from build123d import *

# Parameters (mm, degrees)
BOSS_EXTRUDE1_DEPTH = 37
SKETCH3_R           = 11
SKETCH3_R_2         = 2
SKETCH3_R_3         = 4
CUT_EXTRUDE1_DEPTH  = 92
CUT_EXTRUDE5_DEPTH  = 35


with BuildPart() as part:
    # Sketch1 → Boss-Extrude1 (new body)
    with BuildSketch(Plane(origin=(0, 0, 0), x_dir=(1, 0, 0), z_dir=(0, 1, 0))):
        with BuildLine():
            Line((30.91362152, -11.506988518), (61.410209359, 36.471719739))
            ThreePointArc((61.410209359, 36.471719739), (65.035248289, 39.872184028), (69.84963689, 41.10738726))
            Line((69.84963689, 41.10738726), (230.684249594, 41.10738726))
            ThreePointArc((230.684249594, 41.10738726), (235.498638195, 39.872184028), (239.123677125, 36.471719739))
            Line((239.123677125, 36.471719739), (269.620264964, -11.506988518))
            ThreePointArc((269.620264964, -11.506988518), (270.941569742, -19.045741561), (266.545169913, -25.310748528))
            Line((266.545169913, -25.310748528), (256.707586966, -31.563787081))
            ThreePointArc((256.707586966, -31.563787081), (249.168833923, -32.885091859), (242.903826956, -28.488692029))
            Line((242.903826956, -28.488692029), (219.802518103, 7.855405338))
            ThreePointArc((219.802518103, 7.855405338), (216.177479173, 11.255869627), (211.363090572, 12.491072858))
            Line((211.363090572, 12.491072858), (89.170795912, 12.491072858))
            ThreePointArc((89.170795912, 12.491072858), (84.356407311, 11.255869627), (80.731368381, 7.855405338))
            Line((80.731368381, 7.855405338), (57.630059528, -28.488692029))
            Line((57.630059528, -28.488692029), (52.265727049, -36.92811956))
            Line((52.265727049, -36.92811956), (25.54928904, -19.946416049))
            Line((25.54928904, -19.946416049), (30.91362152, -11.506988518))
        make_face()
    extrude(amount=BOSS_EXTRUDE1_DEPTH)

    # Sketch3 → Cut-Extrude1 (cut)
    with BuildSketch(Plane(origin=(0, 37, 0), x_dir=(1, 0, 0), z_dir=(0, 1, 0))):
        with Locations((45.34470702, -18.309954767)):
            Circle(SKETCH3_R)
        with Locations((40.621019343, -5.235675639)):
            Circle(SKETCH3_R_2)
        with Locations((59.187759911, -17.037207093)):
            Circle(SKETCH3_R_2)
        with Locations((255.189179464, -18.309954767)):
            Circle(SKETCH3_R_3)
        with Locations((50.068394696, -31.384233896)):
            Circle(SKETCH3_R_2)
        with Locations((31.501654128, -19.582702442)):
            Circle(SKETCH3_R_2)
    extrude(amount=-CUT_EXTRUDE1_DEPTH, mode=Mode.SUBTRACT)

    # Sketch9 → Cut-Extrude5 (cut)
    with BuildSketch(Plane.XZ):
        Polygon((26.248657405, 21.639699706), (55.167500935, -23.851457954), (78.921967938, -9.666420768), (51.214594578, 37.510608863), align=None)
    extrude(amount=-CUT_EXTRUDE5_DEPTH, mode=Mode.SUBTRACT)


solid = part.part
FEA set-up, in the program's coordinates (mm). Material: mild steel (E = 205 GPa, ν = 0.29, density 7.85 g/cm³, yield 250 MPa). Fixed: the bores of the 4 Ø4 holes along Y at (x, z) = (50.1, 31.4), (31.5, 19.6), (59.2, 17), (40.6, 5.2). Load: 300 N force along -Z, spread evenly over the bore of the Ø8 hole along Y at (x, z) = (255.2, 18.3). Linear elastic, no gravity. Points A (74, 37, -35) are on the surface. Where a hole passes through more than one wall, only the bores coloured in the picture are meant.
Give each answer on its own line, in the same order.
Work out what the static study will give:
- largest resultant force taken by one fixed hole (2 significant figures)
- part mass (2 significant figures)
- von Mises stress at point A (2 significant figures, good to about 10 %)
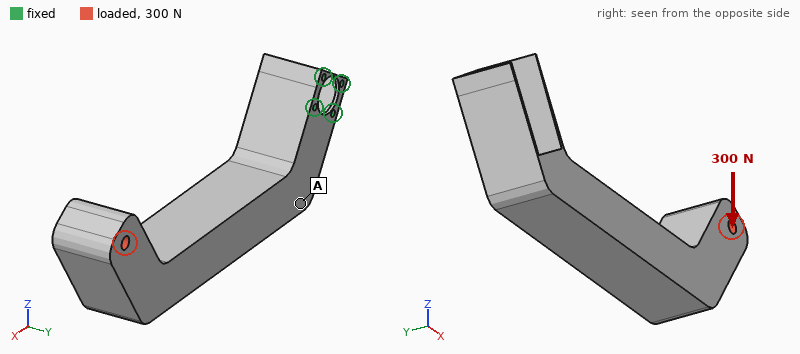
2.1 kN
2.0 kg
12 MPa
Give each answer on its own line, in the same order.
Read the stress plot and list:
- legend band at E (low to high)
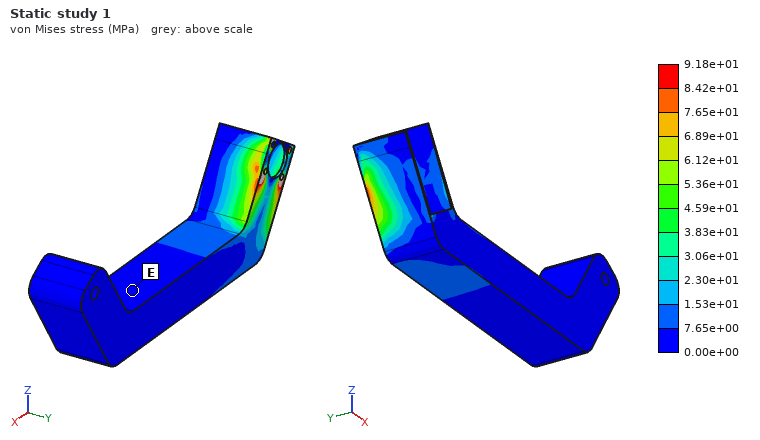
0.00e+00 to 7.65e+00 MPa
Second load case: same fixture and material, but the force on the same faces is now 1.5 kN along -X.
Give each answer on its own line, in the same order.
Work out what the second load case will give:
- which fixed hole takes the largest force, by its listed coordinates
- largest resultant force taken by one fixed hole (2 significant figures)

(59.2, 17)
1.5 kN
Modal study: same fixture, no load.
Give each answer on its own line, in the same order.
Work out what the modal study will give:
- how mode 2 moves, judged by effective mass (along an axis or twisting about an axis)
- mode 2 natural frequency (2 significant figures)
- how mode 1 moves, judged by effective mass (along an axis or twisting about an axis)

along Z
220 Hz
along Y
